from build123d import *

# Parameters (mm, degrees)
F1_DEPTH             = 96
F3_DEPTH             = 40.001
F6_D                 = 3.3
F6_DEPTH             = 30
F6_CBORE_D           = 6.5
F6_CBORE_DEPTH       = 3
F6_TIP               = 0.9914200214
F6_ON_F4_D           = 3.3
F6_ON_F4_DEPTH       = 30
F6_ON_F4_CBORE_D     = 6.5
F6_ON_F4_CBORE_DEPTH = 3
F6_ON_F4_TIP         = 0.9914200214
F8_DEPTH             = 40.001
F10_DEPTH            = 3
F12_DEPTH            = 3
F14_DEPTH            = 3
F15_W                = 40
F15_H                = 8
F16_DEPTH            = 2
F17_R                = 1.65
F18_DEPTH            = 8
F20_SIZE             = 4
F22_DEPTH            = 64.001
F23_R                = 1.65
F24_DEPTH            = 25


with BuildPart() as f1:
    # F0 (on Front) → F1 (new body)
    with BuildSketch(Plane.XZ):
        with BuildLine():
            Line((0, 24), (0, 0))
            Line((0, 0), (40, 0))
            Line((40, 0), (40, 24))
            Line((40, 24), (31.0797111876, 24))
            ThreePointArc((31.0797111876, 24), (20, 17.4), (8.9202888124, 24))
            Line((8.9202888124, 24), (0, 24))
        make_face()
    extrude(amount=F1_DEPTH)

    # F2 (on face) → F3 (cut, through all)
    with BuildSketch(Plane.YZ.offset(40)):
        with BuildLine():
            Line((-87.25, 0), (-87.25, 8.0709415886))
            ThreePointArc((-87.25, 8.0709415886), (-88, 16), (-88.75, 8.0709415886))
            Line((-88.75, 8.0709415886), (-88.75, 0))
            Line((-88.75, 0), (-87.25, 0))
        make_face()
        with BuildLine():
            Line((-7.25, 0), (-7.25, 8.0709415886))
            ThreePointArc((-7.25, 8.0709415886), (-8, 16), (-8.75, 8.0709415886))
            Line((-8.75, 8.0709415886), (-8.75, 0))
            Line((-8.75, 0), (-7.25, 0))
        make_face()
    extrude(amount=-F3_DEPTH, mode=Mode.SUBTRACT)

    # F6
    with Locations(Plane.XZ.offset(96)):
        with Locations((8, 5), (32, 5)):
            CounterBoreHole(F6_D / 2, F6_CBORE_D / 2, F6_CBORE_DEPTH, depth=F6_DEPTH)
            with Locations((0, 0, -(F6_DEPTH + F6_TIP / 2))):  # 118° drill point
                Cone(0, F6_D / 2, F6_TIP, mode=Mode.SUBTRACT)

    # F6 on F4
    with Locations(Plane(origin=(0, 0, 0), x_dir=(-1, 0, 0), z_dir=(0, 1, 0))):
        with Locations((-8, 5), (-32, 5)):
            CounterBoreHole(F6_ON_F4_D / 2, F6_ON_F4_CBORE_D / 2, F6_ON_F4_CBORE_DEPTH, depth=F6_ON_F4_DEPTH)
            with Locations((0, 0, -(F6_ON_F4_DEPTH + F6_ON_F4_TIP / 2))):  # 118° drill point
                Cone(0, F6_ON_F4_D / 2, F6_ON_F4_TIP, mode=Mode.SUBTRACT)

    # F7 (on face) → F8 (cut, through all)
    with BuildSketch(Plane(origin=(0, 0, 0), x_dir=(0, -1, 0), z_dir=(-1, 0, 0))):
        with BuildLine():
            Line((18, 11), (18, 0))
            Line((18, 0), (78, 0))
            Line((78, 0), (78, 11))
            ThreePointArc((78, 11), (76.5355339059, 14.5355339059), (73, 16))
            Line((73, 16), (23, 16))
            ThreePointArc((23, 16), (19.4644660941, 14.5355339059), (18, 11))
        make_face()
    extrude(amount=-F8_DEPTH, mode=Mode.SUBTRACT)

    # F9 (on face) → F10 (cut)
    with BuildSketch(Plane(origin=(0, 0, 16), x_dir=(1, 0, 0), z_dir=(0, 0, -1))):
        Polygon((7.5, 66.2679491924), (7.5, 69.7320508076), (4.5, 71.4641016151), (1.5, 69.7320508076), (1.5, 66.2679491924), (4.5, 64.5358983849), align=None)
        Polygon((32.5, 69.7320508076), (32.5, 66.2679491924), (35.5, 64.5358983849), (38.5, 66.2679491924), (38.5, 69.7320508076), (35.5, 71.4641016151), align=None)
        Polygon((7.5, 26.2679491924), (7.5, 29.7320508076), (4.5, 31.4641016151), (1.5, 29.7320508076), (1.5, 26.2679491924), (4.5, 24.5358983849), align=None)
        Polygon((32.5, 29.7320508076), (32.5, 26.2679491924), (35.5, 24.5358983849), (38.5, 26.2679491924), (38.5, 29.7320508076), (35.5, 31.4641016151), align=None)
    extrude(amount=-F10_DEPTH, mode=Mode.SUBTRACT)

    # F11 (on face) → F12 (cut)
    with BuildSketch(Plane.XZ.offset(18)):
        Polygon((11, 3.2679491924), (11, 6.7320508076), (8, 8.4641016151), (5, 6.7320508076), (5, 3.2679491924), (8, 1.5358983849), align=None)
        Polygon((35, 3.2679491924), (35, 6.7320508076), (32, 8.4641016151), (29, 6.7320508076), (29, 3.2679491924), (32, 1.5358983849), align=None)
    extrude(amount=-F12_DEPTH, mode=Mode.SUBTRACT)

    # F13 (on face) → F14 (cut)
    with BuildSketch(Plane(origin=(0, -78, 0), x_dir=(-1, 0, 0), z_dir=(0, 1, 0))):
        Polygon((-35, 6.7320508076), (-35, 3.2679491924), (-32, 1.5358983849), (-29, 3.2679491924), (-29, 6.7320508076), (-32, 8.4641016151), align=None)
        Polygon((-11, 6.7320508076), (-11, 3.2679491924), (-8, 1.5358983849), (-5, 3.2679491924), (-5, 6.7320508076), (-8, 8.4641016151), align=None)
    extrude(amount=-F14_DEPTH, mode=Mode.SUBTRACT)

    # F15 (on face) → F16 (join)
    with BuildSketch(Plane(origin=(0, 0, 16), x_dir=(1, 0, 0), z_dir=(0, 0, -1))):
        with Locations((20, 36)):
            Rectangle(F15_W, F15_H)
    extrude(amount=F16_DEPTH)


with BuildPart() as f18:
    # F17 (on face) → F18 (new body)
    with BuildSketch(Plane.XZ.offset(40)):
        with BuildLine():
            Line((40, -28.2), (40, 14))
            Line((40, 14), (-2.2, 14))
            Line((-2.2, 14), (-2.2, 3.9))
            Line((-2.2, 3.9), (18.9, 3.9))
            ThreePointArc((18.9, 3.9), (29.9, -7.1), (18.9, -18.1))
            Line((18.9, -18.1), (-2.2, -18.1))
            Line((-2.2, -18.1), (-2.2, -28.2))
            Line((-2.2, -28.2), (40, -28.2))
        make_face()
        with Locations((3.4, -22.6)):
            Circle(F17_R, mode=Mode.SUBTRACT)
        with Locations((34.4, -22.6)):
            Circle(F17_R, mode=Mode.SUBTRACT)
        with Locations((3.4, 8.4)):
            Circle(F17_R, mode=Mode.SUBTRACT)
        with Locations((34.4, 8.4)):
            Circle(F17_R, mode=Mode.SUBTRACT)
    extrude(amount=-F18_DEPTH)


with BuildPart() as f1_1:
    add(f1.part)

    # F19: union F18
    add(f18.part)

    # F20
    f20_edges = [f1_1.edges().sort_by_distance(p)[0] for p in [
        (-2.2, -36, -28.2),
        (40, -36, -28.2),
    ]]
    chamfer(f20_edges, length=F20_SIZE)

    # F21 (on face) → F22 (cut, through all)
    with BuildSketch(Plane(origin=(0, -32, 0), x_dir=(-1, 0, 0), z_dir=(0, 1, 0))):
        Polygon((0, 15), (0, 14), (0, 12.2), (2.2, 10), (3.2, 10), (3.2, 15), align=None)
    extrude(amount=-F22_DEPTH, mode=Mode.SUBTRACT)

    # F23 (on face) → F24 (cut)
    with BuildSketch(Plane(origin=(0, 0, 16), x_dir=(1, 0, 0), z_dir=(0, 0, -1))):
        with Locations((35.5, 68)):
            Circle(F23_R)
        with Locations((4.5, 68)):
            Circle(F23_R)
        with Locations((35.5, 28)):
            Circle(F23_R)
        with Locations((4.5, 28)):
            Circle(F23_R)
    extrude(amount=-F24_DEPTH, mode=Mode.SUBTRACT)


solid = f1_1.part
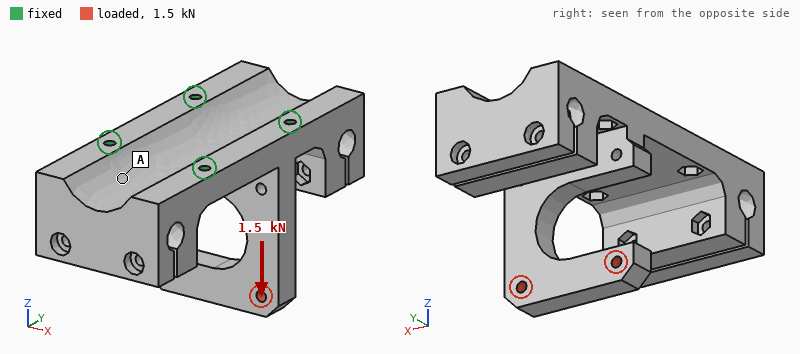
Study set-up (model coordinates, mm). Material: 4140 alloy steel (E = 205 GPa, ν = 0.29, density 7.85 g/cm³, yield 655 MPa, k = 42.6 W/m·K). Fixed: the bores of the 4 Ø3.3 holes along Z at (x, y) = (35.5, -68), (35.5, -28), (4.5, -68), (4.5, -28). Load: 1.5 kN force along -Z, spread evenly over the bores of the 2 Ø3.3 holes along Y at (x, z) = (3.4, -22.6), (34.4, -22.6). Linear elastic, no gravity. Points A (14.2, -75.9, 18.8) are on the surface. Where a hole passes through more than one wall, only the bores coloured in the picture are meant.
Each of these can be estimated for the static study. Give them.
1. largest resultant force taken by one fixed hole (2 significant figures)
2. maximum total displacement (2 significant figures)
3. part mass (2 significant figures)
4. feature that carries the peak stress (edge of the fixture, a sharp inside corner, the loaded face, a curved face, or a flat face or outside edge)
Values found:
890 N
0.17 mm
370 g
a curved face
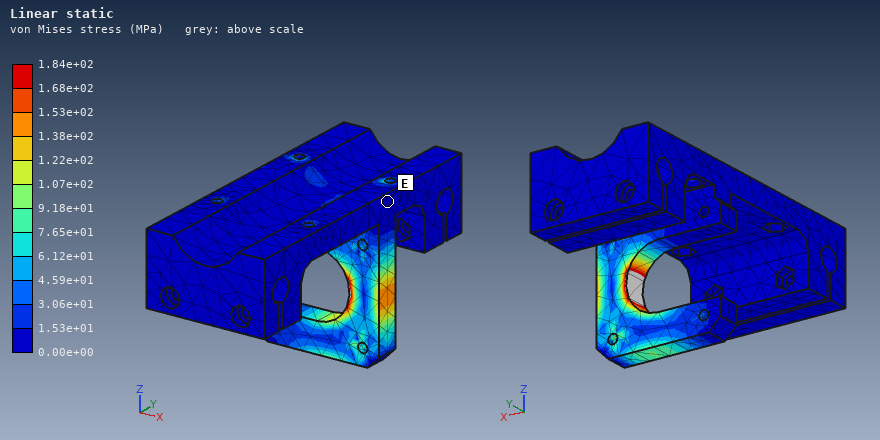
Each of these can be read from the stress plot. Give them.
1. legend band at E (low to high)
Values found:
0.00e+00 to 1.53e+01 MPa
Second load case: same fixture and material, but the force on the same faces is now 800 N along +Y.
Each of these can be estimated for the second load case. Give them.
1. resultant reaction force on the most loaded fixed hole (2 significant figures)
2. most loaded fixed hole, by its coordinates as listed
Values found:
890 N
(35.5, -68)
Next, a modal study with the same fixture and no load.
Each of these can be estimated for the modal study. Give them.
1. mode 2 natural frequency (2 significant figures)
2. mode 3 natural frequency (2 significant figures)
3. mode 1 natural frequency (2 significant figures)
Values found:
2900 Hz
3100 Hz
1700 Hz
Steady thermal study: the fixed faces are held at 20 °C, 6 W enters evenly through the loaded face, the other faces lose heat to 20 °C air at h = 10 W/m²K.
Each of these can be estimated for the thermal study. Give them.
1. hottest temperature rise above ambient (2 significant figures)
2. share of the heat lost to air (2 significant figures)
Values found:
67 K
23 %
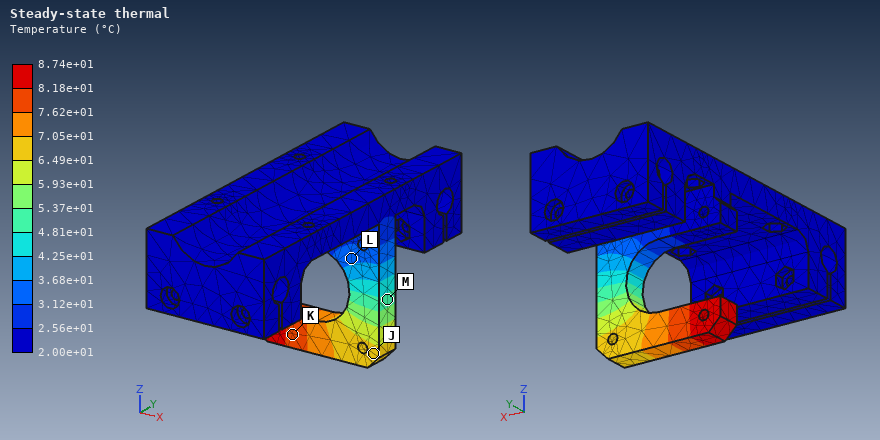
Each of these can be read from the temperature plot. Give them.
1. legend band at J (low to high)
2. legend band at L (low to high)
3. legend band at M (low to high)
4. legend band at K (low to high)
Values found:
6.49e+01 to 7.05e+01 °C
3.12e+01 to 3.68e+01 °C
4.81e+01 to 5.37e+01 °C
7.62e+01 to 8.18e+01 °C
